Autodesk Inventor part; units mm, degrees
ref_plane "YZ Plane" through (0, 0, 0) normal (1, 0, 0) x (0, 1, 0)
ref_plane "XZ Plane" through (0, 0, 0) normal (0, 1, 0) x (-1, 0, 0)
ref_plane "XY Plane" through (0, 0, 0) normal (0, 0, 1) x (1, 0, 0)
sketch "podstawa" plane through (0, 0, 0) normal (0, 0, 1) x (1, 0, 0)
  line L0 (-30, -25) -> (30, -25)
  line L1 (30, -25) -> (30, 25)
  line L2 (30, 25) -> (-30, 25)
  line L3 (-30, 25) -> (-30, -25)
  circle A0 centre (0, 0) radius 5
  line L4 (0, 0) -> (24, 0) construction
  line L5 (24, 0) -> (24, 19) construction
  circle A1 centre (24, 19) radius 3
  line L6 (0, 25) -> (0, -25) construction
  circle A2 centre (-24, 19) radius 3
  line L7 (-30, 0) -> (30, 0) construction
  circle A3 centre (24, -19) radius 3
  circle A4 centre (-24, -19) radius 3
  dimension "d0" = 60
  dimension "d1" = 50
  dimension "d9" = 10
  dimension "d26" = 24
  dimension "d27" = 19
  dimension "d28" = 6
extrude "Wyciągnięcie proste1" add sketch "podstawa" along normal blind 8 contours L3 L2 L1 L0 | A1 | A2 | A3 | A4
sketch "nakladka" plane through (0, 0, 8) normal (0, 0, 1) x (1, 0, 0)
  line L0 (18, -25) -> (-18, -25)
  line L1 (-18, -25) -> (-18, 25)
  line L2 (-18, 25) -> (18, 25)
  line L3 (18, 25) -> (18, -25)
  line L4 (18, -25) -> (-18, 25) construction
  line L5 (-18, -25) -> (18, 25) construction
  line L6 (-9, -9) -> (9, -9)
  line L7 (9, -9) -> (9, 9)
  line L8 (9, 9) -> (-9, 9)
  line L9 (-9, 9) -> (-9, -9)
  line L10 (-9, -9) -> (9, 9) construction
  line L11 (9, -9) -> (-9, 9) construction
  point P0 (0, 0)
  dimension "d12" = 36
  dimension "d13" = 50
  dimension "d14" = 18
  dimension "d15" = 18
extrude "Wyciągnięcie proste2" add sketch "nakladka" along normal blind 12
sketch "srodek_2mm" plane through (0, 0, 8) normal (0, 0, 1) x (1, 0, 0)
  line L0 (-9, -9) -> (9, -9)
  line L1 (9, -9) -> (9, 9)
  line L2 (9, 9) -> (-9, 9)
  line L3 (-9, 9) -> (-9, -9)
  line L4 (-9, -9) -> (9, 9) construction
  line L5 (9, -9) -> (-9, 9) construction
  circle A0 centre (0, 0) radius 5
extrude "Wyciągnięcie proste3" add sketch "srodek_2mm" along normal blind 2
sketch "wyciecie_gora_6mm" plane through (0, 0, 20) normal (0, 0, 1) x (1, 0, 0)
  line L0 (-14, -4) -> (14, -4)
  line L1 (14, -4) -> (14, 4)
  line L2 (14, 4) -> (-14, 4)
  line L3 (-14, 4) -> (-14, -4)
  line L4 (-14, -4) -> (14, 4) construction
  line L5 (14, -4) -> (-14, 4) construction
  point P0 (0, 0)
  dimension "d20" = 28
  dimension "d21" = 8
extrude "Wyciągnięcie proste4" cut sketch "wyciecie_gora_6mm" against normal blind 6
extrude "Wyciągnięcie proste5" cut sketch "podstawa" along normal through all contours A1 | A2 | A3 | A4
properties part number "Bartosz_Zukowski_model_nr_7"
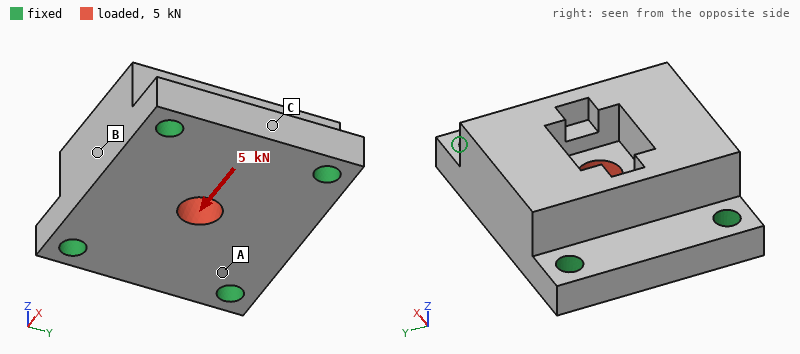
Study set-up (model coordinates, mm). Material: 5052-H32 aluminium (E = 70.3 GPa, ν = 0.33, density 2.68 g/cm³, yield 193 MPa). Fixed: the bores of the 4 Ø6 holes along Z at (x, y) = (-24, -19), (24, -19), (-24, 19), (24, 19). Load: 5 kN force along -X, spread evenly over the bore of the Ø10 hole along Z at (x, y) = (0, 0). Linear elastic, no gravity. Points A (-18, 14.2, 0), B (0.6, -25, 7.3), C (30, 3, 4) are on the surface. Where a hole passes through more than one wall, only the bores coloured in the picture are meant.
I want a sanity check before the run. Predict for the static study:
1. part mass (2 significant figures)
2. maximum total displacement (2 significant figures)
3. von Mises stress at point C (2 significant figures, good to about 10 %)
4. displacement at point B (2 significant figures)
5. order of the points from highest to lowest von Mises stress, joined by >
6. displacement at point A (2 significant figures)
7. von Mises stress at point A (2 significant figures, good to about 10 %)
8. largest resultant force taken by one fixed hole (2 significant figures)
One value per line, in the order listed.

110 g
4.8 µm
6.1 MPa
1.2 µm
A > C > B
1.1 µm
12 MPa
1.3 kN
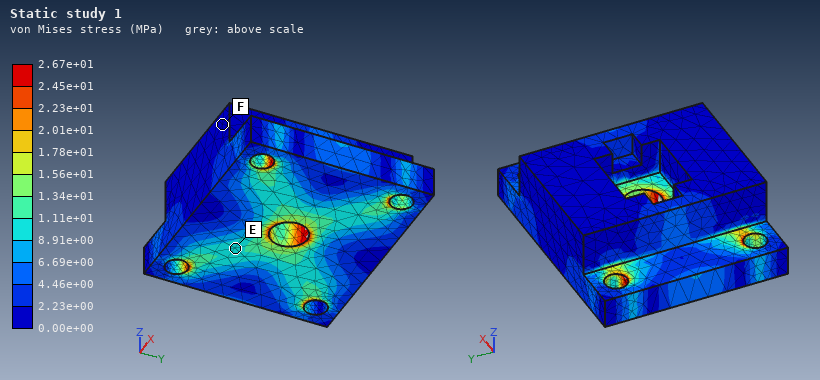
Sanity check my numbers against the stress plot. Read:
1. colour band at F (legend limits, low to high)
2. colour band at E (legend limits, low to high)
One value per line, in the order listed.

0.00e+00 to 2.23e+00 MPa
8.91e+00 to 1.11e+01 MPa
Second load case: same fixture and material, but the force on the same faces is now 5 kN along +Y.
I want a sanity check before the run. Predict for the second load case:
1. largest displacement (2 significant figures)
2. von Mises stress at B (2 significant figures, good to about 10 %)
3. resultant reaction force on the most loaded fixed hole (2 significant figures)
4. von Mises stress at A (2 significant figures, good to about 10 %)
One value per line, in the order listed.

6.1 µm
6.6 MPa
1.4 kN
14 MPa
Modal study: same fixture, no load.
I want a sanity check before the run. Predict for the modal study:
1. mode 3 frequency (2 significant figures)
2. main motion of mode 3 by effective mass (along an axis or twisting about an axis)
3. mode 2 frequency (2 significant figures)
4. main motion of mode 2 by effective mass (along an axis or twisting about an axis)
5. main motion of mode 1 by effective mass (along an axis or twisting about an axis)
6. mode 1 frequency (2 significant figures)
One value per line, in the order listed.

23 kHz
along Y
17 kHz
along Y
along Z
16 kHz
